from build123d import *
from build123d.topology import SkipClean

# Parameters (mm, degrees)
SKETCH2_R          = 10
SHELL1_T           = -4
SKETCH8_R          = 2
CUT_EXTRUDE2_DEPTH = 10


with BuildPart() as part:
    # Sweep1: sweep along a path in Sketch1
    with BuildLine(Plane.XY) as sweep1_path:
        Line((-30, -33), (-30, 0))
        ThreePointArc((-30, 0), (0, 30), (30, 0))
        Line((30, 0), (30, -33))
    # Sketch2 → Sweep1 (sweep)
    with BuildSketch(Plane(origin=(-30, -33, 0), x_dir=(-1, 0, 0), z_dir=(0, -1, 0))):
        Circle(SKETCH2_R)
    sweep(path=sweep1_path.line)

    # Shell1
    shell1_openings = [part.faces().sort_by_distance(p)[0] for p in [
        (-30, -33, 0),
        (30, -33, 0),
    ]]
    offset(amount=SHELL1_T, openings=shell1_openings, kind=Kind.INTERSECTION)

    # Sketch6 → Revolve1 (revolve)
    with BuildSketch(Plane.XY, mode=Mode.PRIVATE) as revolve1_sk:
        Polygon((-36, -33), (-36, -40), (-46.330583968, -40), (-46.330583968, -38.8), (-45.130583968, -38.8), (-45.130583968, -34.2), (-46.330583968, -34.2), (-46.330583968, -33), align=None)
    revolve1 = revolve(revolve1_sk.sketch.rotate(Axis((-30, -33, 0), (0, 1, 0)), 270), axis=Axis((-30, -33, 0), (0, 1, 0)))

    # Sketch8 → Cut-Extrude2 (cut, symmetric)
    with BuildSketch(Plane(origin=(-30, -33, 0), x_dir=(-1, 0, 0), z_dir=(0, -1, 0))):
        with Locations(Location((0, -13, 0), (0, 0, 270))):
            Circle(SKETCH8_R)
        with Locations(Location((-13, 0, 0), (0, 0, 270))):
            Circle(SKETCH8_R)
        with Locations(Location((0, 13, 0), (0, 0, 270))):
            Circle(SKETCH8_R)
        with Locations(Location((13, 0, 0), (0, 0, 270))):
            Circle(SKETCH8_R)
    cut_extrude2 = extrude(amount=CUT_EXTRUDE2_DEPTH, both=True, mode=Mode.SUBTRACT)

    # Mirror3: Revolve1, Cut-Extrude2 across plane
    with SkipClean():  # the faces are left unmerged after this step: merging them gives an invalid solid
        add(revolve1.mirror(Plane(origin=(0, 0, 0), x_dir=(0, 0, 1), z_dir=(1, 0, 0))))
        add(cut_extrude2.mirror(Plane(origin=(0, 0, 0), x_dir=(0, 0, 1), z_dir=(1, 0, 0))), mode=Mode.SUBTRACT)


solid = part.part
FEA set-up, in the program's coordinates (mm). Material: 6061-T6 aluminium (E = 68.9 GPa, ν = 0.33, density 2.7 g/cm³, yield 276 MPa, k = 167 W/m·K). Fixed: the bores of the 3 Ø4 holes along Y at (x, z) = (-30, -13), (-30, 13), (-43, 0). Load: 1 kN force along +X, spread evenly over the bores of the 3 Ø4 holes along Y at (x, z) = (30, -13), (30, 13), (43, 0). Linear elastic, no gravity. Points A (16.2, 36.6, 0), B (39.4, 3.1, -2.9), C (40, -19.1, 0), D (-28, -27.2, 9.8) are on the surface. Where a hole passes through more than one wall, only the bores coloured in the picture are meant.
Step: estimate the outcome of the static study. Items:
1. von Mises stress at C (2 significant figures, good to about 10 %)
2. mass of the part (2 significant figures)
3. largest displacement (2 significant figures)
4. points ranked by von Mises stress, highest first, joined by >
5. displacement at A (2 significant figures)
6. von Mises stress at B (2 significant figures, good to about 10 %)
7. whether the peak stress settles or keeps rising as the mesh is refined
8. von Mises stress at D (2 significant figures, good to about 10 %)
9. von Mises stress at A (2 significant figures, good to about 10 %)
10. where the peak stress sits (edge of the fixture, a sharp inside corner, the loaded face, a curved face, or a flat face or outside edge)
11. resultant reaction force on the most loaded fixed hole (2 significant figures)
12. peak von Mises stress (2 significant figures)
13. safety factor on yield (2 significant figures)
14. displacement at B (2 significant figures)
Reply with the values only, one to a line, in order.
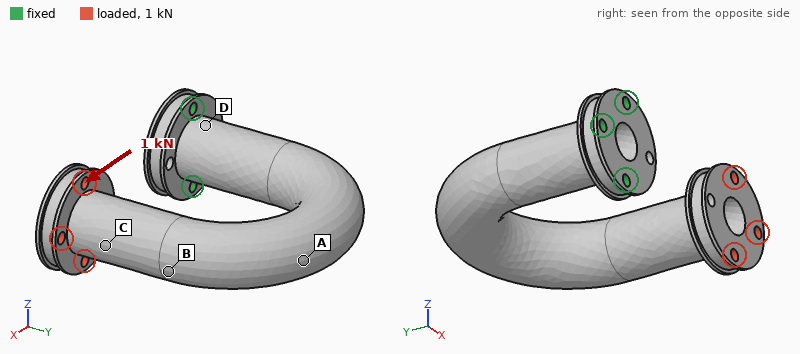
28 MPa
110 g
1.2 mm
A > B > C > D
0.36 mm
51 MPa
settles
14 MPa
83 MPa
a curved face
380 N
130 MPa
2.1
0.66 mm
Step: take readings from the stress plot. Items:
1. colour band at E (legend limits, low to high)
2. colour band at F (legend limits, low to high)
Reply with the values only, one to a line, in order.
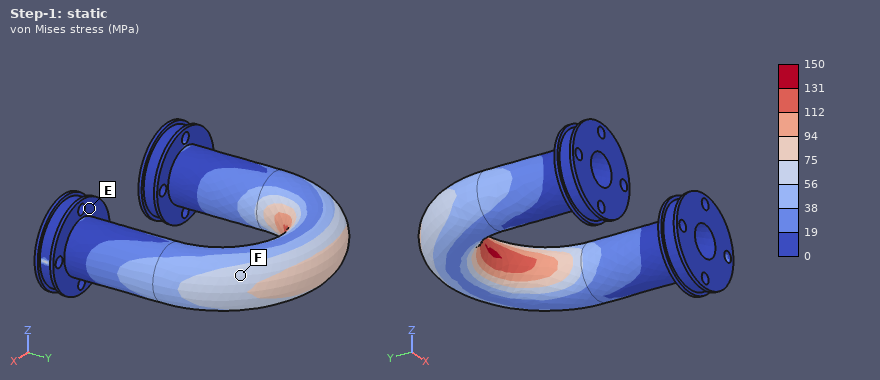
0 to 19 MPa
56 to 75 MPa
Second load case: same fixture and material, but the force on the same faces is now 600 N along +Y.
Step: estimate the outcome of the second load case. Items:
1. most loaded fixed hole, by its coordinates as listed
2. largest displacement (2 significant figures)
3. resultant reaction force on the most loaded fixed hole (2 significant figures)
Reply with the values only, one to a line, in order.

(-43, 0)
0.72 mm
2.0 kN
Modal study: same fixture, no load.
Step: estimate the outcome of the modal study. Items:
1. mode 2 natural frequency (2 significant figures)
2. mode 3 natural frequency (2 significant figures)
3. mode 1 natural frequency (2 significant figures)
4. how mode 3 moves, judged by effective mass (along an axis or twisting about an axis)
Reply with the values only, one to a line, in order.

720 Hz
1300 Hz
720 Hz
along X
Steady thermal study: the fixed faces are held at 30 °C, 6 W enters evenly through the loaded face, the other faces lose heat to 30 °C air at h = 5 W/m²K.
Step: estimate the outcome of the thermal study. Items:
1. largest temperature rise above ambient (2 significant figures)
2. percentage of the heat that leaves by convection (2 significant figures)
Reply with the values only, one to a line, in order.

26 K
21 %
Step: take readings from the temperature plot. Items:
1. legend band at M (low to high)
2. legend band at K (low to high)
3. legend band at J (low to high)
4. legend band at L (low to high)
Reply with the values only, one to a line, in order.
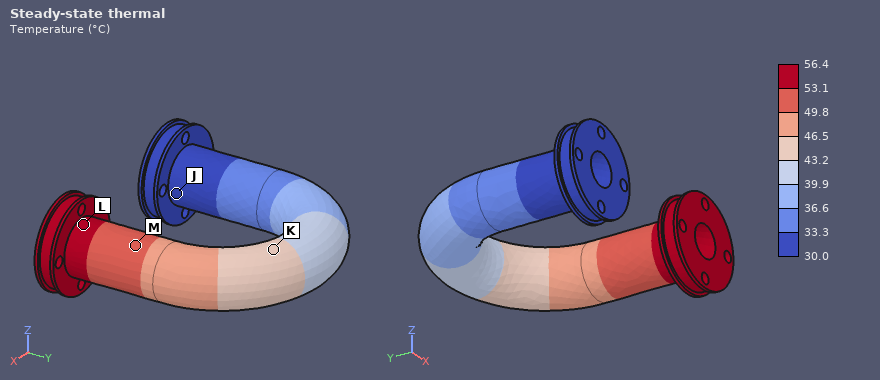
49.8 to 53.1 °C
43.2 to 46.5 °C
30.0 to 33.3 °C
53.1 to 56.4 °C
